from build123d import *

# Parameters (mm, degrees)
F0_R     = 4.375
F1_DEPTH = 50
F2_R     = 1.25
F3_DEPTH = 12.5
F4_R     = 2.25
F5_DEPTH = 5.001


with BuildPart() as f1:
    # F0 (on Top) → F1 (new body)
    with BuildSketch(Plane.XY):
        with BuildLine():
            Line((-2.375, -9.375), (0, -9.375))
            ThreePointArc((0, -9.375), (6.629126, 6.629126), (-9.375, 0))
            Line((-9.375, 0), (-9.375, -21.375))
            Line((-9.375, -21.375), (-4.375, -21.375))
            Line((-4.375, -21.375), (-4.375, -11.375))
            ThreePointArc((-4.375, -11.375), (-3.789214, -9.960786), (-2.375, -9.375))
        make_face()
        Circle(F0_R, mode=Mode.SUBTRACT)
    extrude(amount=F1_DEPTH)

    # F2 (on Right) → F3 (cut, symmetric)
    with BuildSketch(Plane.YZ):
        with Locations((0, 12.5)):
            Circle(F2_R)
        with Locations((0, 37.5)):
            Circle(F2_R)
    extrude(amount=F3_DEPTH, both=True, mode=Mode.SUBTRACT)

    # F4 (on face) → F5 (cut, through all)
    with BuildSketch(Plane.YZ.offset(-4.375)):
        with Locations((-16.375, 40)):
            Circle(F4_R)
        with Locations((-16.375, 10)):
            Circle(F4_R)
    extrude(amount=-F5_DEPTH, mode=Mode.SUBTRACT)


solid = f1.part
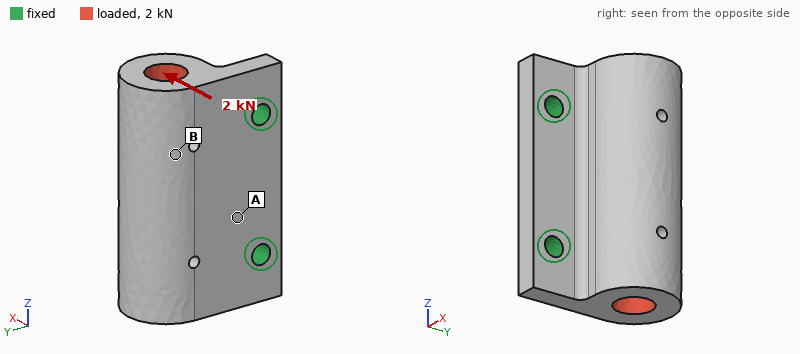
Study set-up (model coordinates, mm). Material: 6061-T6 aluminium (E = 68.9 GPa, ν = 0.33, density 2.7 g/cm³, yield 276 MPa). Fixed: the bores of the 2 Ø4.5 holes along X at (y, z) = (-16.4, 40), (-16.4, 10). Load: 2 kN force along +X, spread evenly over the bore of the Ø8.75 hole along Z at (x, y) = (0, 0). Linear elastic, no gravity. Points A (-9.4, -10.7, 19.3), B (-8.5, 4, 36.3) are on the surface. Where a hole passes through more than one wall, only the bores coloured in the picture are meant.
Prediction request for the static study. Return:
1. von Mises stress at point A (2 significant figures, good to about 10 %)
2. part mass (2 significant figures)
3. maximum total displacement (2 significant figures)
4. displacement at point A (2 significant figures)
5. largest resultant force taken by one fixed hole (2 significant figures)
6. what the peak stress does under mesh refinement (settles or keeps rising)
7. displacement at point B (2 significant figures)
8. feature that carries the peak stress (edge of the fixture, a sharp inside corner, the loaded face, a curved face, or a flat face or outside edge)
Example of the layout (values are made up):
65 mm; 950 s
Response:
63 MPa; 39 g; 0.17 mm; 0.026 mm; 1.0 kN; keeps rising; 0.12 mm; edge of the fixture
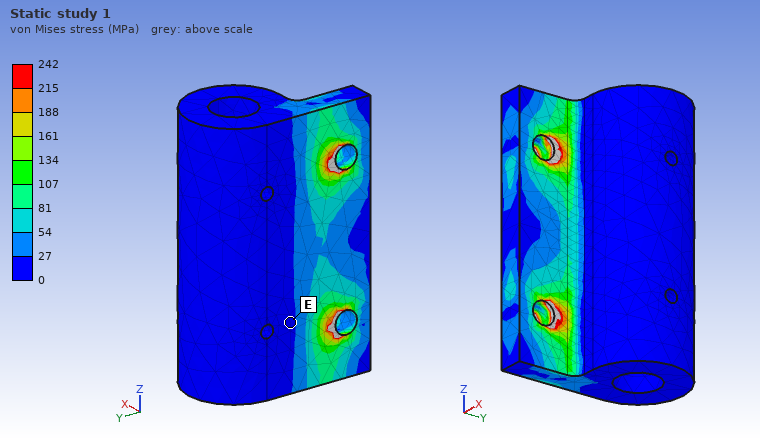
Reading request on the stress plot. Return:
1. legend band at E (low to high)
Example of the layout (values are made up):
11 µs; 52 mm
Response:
0 to 27 MPa
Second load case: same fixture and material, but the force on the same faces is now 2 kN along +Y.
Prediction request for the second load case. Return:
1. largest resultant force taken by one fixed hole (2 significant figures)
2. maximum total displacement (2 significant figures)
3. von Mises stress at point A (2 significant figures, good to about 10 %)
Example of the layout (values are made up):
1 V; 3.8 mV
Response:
1.0 kN; 89 µm; 37 MPa
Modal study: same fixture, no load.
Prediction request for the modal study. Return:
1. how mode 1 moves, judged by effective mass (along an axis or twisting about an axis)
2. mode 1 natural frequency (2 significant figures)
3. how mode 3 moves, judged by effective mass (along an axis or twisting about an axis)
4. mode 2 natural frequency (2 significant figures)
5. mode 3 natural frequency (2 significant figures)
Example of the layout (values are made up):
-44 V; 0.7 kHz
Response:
along X; 3500 Hz; along Z; 10 kHz; 14 kHz
